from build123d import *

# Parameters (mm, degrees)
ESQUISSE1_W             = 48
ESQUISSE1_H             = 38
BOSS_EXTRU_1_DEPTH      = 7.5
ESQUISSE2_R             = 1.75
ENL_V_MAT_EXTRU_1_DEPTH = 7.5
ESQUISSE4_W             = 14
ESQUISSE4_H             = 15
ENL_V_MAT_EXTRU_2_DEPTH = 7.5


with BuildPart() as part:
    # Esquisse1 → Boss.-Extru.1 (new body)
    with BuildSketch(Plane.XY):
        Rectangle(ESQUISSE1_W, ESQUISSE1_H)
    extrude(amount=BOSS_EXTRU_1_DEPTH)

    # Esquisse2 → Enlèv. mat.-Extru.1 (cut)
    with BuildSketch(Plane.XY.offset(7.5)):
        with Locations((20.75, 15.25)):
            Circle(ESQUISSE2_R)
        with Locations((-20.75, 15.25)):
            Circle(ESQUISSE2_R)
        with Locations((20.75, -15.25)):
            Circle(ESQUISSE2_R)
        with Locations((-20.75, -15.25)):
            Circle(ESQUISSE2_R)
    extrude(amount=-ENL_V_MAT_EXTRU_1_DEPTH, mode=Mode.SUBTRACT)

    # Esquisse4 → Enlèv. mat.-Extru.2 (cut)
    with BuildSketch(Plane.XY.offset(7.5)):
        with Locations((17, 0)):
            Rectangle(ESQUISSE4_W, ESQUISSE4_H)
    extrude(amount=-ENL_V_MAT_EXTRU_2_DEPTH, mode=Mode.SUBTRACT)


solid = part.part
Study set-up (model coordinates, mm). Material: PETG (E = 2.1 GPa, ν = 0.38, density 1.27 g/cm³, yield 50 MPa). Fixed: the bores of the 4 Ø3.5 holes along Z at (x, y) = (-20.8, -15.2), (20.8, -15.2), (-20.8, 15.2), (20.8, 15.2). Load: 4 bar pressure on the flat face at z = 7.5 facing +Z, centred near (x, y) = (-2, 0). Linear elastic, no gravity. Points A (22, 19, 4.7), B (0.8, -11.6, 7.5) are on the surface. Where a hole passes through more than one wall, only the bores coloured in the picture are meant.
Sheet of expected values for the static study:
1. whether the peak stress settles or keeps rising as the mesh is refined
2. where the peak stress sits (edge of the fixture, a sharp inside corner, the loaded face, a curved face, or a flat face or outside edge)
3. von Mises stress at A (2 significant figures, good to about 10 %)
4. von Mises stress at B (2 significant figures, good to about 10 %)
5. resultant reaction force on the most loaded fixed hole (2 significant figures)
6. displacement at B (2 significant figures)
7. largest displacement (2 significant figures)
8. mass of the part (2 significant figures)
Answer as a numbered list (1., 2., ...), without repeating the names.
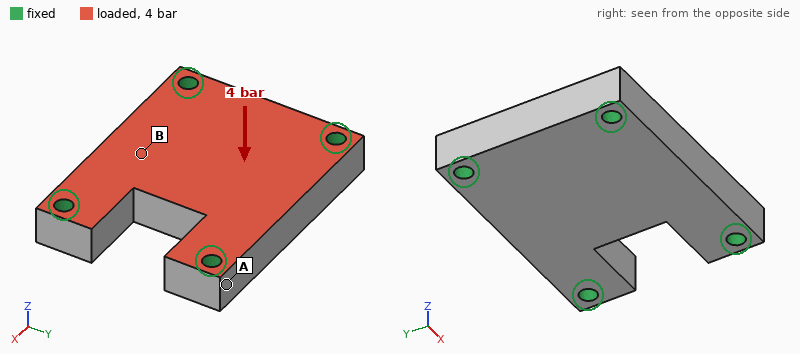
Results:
1. keeps rising
2. edge of the fixture
3. 1.3 MPa
4. 3.3 MPa
5. 180 N
6. 80 µm
7. 90 µm
8. 15 g
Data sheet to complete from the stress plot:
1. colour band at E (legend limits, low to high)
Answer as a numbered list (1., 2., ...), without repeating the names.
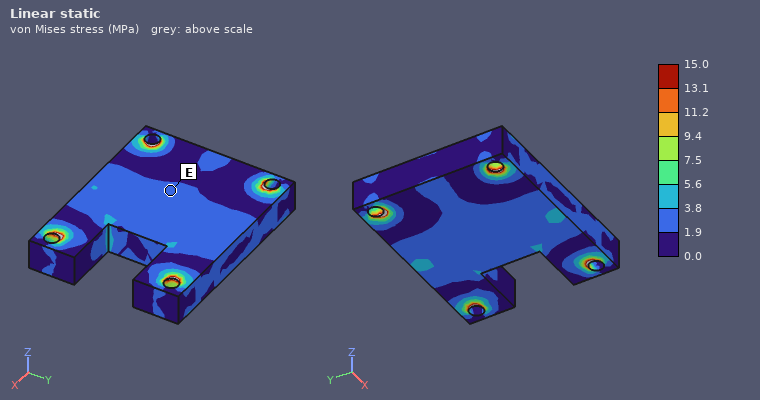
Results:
1. 1.9 to 3.8 MPa
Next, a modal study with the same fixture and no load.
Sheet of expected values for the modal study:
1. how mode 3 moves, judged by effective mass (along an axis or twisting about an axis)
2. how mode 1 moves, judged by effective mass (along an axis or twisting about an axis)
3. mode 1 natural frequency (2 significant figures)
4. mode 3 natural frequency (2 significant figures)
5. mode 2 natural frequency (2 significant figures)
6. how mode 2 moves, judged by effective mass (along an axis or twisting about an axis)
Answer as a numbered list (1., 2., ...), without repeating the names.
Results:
1. along Y
2. along Z
3. 3900 Hz
4. 6300 Hz
5. 5500 Hz
6. twisting about X
